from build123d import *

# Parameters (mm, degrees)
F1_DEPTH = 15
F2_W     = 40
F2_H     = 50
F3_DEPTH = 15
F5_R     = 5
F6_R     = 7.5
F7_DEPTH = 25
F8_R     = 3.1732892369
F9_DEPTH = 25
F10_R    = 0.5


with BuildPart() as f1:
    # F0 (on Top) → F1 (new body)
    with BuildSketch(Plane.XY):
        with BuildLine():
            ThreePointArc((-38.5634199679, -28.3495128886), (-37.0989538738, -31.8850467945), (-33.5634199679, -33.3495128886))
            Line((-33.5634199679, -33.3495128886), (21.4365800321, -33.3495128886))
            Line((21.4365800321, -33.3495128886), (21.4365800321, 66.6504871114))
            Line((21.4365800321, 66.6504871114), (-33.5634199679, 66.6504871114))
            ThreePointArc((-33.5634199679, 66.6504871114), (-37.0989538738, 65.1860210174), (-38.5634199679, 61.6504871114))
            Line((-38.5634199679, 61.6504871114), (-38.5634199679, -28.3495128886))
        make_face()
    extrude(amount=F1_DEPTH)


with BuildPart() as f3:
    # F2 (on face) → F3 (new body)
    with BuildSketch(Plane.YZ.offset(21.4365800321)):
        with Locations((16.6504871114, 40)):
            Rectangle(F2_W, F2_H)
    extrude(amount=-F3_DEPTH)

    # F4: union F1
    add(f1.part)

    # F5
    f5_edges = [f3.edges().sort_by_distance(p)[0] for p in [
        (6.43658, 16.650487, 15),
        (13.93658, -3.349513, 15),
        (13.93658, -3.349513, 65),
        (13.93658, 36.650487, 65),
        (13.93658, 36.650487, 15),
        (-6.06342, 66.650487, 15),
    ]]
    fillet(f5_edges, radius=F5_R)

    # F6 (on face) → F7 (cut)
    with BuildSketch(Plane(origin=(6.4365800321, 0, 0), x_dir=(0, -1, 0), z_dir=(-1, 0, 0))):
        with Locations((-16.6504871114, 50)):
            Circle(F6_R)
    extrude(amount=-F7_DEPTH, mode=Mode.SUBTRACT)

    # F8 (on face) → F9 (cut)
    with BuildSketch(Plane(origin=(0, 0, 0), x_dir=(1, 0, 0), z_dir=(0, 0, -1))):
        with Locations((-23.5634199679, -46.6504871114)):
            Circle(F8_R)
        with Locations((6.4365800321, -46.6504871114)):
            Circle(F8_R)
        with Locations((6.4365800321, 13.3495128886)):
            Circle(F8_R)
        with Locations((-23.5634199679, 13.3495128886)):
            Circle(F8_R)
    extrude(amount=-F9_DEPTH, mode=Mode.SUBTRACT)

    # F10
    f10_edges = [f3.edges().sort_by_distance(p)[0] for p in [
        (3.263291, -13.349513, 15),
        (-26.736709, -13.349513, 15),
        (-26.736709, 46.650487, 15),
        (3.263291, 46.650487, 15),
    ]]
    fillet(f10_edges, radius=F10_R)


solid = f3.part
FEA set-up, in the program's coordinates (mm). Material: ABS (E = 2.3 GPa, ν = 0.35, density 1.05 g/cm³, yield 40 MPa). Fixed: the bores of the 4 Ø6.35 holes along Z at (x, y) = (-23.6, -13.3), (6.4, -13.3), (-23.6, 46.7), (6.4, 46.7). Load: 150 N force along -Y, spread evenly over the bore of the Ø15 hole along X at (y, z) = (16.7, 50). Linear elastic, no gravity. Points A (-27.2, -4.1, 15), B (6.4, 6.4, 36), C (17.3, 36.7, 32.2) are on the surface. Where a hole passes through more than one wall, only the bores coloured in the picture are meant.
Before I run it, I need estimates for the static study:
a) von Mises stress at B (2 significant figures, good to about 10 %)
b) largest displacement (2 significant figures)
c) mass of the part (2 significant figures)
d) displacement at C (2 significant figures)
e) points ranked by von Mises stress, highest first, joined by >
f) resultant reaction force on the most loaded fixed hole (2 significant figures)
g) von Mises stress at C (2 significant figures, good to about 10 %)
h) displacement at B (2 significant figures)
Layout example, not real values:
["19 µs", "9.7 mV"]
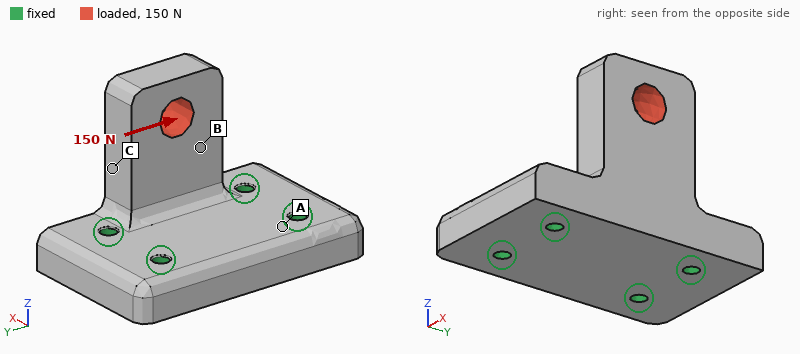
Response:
["0.47 MPa", "63 µm", "120 g", "25 µm", "C > B > A", "140 N", "0.75 MPa", "25 µm"]
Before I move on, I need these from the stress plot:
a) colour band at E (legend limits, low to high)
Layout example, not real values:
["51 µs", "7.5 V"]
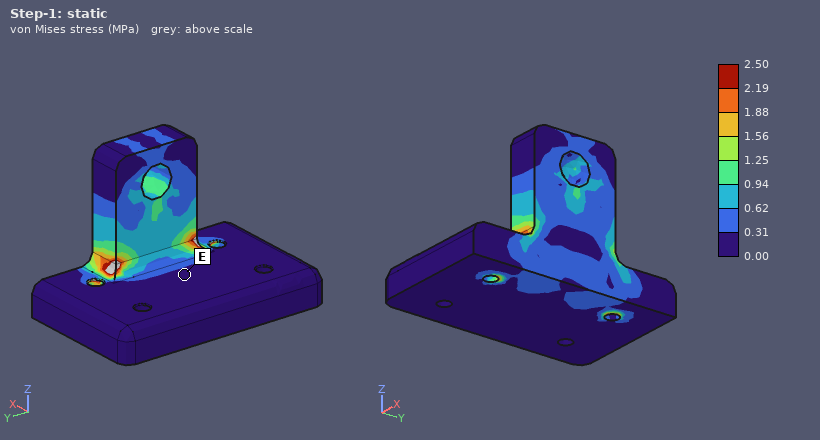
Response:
["0.00 to 0.31 MPa"]
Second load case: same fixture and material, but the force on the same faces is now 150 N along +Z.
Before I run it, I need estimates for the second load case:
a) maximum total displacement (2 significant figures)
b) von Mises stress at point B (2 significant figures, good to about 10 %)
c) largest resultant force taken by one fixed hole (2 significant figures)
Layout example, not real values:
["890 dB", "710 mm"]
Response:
["28 µm", "0.30 MPa", "82 N"]
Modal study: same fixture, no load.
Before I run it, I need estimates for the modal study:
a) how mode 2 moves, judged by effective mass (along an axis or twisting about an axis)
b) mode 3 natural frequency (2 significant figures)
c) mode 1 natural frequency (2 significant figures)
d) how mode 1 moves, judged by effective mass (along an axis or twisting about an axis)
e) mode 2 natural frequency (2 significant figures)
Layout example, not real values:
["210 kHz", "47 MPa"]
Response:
["along Y", "2800 Hz", "1000 Hz", "along X", "2100 Hz"]
